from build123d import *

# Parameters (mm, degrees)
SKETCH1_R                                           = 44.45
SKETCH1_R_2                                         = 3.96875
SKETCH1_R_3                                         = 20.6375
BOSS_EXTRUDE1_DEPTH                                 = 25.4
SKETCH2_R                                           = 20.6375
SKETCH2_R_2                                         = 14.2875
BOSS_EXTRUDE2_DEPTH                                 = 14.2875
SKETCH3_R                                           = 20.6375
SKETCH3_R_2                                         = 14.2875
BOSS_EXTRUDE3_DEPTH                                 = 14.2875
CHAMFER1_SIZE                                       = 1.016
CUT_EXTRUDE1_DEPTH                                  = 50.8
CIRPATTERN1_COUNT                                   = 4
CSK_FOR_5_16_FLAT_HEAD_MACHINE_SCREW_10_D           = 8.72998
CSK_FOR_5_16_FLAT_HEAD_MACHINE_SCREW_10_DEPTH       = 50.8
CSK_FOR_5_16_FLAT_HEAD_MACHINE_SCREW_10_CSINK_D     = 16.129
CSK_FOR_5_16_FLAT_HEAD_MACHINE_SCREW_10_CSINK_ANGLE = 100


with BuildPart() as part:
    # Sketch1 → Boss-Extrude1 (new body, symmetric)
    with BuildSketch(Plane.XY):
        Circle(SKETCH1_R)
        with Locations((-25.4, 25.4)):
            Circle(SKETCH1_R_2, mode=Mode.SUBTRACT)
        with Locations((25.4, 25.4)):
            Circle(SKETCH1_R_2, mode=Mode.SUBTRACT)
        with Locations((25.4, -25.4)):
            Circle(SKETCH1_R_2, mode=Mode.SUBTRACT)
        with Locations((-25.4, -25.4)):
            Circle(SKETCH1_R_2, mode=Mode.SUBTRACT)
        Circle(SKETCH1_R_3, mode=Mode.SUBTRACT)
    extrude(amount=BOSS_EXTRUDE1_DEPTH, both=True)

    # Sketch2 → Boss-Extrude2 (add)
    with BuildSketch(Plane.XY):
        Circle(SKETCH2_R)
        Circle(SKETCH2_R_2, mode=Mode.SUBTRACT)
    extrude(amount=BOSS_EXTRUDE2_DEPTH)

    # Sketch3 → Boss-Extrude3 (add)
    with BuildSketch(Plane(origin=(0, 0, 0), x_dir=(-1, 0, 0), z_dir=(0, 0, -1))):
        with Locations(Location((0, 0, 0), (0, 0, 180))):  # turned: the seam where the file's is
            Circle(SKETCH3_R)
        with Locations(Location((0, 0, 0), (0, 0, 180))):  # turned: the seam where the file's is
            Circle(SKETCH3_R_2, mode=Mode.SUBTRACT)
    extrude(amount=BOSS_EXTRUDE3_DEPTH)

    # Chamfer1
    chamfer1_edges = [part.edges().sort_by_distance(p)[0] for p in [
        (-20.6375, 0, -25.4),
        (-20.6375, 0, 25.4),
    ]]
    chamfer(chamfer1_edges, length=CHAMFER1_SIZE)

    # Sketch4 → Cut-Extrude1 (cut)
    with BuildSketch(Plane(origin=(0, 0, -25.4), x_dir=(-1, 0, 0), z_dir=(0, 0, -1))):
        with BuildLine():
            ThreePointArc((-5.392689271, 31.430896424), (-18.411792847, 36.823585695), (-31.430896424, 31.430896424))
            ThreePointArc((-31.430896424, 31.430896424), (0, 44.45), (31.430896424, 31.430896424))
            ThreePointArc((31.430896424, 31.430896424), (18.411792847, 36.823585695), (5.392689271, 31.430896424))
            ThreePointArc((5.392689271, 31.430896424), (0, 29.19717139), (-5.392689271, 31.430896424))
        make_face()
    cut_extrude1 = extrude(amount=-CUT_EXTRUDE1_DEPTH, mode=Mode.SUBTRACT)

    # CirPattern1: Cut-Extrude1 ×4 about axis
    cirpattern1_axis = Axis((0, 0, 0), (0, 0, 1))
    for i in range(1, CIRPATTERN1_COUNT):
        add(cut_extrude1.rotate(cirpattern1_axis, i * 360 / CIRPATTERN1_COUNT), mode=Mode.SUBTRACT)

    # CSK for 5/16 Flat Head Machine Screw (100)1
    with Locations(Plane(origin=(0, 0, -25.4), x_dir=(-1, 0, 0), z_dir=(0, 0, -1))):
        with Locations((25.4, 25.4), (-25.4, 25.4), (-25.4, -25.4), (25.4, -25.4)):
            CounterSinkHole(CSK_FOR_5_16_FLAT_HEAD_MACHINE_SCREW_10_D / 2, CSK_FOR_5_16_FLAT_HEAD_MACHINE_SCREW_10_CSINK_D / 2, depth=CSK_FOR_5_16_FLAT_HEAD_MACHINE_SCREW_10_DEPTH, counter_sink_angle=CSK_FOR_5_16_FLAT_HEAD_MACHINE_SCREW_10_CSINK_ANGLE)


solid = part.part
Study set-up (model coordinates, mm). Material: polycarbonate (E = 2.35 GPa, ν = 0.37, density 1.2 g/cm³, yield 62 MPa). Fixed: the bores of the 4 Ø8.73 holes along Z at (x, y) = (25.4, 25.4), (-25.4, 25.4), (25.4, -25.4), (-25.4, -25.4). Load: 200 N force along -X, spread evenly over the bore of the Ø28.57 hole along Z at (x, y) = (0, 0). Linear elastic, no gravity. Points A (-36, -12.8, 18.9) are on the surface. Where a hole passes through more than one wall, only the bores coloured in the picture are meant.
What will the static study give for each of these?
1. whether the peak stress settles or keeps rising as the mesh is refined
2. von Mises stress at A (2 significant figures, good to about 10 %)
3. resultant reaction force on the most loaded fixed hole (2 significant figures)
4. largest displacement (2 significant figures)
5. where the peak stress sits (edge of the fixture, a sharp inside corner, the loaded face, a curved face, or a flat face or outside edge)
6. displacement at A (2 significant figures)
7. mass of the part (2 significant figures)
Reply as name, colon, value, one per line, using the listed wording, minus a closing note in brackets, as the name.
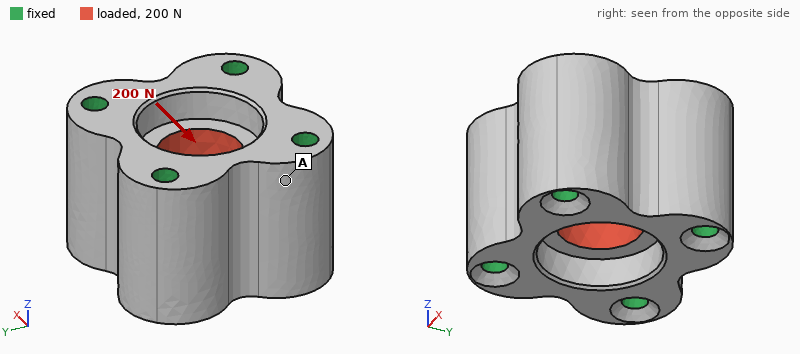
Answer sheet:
whether the peak stress settles or keeps rising as the mesh is refined: keeps rising
von Mises stress at A: 0.021 MPa
resultant reaction force on the most loaded fixed hole: 56 N
largest displacement: 1.3 µm
where the peak stress sits: edge of the fixture
displacement at A: 0.55 µm
mass of the part: 210 g
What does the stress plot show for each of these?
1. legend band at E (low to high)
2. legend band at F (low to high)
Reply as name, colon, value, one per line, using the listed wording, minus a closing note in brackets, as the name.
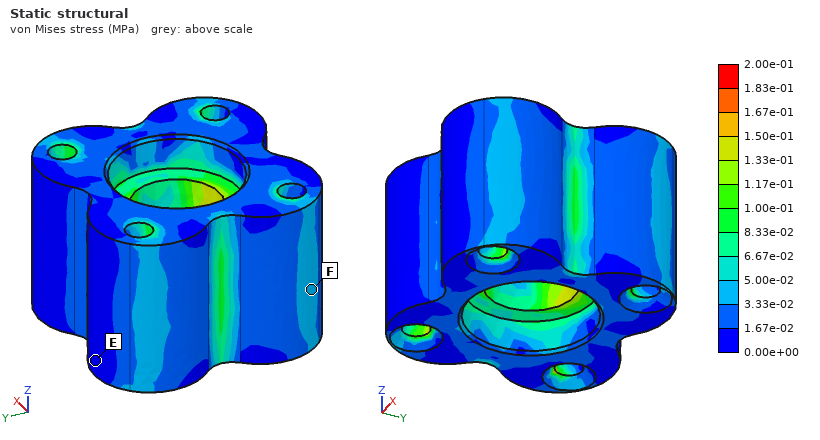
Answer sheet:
legend band at E: 0.00e+00 to 1.67e-02 MPa
legend band at F: 3.33e-02 to 5.00e-02 MPa
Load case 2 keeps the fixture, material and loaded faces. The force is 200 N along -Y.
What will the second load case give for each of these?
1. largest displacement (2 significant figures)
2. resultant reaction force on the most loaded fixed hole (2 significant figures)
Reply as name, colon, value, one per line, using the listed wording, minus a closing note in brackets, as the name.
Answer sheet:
largest displacement: 1.3 µm
resultant reaction force on the most loaded fixed hole: 56 N
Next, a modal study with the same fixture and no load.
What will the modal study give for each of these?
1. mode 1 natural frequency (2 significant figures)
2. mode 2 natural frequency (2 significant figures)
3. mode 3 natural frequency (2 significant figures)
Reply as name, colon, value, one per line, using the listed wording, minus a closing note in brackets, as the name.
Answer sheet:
mode 1 natural frequency: 5900 Hz
mode 2 natural frequency: 7900 Hz
mode 3 natural frequency: 7900 Hz
